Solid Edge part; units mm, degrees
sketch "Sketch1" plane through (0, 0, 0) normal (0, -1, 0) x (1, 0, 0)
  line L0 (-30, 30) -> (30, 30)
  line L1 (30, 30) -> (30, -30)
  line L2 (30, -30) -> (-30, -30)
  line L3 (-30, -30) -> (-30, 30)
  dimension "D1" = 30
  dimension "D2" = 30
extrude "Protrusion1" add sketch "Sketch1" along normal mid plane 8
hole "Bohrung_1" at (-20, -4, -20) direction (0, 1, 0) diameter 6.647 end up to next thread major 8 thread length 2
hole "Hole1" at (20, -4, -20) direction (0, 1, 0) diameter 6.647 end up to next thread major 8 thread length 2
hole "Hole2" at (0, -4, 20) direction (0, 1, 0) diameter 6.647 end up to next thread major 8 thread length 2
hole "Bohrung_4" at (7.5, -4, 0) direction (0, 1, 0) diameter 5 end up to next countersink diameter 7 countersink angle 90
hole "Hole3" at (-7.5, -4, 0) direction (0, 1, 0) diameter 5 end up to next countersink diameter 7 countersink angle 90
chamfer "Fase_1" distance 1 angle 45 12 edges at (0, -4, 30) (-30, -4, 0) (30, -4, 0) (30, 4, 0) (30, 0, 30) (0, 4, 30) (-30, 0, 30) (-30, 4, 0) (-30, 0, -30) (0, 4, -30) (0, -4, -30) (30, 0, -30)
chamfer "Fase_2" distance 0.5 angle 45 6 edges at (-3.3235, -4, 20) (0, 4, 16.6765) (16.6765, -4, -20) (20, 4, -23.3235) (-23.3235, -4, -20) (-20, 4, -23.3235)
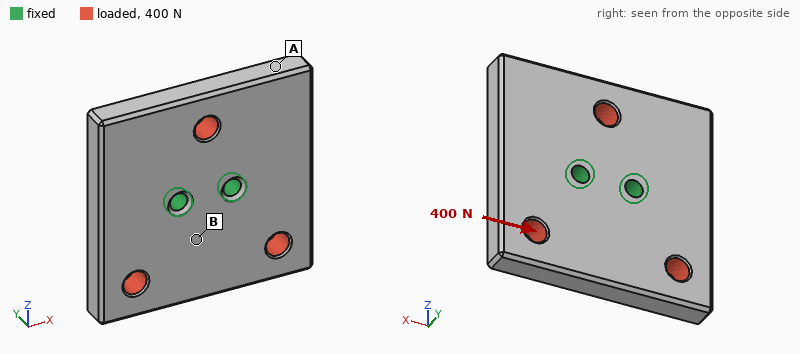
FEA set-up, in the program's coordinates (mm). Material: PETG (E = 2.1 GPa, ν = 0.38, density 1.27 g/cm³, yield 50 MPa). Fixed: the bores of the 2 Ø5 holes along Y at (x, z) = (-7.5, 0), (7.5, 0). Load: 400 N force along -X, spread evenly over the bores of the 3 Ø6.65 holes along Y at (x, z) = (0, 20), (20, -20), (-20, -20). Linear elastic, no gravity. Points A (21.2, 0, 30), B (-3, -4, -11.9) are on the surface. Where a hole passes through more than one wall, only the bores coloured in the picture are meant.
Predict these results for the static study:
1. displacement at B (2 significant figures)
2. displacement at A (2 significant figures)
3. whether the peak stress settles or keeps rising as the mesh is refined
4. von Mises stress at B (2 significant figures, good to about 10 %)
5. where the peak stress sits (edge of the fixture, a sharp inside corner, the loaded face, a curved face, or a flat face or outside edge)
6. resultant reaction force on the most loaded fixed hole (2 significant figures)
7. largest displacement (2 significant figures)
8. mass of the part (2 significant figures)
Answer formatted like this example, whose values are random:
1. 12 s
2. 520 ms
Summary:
1. 18 µm
2. 13 µm
3. keeps rising
4. 1.6 MPa
5. edge of the fixture
6. 240 N
7. 51 µm
8. 35 g
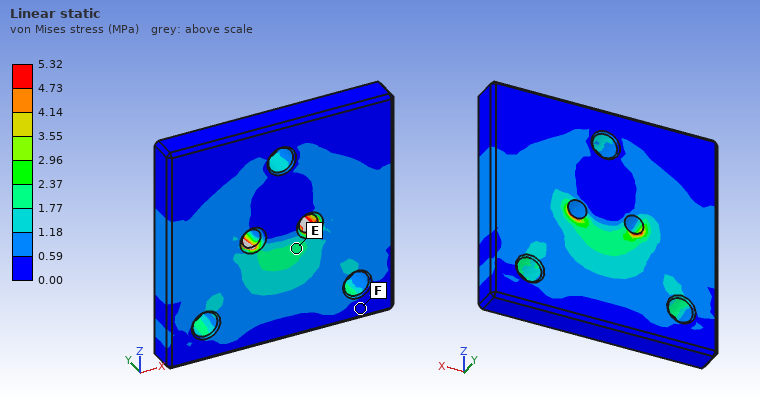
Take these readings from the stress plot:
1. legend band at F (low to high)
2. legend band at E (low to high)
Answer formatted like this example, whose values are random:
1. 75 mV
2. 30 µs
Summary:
1. 0.00 to 0.59 MPa
2. 1.77 to 2.37 MPa
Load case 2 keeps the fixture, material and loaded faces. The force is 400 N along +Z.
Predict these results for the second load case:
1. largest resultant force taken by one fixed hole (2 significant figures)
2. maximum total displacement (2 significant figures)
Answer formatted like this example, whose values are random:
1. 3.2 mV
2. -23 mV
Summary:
1. 200 N
2. 19 µm
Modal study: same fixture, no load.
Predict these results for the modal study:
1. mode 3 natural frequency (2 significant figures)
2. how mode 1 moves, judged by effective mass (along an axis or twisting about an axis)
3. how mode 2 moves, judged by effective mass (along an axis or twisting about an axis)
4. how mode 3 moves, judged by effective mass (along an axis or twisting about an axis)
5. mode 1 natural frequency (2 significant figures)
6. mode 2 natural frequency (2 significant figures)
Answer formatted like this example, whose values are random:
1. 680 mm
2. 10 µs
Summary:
1. 1800 Hz
2. twisting about X
3. twisting about Z
4. along Y
5. 1300 Hz
6. 1800 Hz
